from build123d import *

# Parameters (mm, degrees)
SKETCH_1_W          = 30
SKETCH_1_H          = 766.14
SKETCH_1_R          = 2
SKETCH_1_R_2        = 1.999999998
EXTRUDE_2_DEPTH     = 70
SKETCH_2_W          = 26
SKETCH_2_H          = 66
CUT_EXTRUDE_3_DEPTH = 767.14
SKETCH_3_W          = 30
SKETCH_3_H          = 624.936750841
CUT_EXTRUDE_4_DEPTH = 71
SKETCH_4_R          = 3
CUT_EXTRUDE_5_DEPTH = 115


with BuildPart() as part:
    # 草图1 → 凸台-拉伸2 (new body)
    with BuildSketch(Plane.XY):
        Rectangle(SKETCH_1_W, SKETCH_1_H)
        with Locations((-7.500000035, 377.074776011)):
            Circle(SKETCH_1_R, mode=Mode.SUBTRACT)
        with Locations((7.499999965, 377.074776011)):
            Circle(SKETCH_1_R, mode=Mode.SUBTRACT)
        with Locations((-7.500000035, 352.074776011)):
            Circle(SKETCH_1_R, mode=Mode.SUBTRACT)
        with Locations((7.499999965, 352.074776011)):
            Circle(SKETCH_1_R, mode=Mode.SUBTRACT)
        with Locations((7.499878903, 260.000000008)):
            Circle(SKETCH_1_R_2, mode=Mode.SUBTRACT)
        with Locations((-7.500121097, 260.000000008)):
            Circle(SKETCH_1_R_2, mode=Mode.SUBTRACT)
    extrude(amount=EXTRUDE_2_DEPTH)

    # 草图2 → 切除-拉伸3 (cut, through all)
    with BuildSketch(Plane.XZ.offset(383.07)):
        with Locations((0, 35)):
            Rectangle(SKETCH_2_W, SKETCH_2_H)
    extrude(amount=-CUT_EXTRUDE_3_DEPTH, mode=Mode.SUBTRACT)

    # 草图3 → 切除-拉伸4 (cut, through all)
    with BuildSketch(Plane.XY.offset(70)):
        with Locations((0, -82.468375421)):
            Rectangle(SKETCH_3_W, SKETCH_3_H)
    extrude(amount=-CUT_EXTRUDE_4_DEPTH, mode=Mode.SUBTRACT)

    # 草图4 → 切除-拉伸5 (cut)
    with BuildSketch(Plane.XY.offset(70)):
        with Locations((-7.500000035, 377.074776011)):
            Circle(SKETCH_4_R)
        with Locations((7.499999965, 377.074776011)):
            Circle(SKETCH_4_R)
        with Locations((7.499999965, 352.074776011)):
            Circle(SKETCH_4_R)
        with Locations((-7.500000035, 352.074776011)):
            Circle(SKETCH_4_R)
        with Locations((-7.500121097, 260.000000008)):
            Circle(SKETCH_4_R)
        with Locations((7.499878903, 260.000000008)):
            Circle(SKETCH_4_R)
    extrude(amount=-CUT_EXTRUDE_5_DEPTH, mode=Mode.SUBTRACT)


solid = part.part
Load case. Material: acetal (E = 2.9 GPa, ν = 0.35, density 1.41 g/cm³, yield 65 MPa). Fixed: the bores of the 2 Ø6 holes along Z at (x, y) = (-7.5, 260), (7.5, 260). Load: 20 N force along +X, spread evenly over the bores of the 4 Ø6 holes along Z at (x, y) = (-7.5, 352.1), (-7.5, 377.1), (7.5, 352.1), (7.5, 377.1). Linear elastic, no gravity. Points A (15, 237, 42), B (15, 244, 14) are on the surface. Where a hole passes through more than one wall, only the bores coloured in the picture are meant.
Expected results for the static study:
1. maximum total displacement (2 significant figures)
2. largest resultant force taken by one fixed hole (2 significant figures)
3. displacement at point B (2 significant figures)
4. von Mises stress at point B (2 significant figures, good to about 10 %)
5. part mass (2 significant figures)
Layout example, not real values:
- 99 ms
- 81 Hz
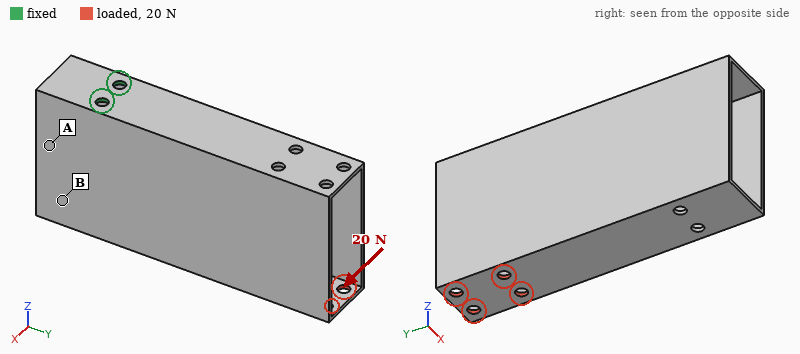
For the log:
- 1.7 mm
- 120 N
- 1.1 mm
- 1.5 MPa
- 82 g
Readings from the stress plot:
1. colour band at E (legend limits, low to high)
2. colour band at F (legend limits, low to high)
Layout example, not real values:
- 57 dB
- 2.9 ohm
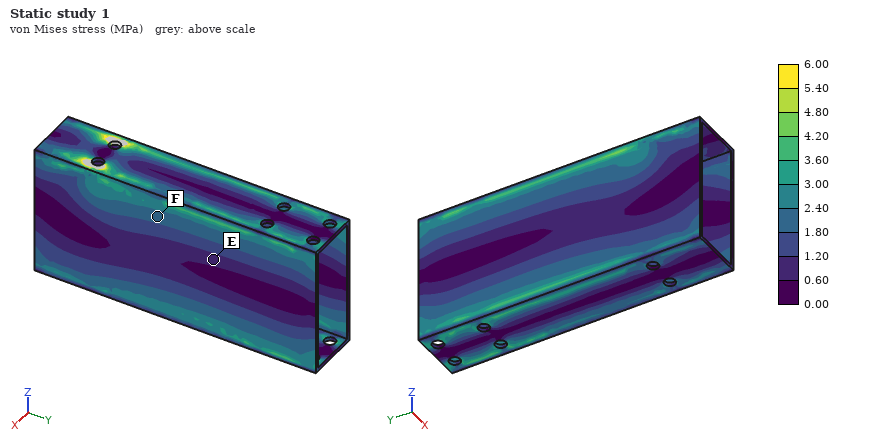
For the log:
- 0.60 to 1.20 MPa
- 1.80 to 2.40 MPa
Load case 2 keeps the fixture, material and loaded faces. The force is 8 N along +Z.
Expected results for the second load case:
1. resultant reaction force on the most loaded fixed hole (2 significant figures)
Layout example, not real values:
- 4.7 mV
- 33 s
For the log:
- 4.0 N
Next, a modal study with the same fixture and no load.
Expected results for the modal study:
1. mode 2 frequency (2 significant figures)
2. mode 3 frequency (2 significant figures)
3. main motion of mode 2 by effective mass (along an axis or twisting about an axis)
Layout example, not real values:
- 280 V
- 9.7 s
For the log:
- 93 Hz
- 210 Hz
- along X
